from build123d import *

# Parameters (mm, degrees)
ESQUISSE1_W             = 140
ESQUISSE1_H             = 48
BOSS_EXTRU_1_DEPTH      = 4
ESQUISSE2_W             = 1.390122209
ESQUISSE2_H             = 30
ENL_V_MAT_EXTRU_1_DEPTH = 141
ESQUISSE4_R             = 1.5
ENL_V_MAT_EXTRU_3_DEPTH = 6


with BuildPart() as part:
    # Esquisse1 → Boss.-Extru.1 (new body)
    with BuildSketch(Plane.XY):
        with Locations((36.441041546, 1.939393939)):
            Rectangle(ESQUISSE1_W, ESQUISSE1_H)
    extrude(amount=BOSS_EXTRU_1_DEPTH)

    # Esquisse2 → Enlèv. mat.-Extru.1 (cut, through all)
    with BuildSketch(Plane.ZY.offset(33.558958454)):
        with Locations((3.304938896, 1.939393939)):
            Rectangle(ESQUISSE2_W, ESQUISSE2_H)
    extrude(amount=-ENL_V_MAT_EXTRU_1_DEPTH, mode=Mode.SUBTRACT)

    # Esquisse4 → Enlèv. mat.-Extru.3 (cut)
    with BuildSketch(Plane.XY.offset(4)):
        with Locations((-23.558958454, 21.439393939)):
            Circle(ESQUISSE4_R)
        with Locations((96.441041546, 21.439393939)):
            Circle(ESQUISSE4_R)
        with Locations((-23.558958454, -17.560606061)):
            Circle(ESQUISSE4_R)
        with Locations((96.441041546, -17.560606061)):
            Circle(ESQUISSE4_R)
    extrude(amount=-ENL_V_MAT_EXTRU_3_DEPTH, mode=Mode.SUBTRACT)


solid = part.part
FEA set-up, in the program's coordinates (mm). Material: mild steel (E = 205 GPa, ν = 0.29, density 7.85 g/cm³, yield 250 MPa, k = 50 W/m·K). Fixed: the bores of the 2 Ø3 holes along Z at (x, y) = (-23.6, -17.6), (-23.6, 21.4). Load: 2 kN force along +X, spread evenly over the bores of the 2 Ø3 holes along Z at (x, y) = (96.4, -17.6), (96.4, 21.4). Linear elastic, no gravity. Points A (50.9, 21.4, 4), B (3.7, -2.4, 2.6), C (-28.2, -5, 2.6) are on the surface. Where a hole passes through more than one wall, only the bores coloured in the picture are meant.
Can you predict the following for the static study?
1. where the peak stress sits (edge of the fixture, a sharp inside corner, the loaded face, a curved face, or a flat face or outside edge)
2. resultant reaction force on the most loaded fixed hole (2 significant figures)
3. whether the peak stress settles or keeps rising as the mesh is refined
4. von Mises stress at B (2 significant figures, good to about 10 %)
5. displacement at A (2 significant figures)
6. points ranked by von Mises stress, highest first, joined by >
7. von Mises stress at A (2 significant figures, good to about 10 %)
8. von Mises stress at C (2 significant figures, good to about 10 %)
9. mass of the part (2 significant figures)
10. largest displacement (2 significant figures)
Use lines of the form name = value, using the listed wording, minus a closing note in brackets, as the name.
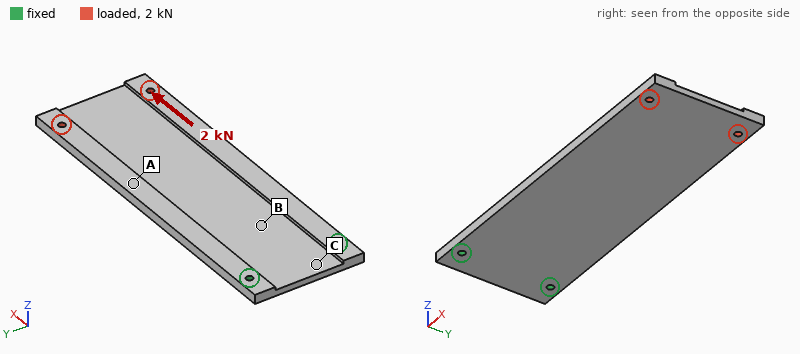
where the peak stress sits = edge of the fixture
resultant reaction force on the most loaded fixed hole = 1.0 kN
whether the peak stress settles or keeps rising as the mesh is refined = keeps rising
von Mises stress at B = 15 MPa
displacement at A = 0.050 mm
points ranked by von Mises stress, highest first, joined by > = A > B > C
von Mises stress at A = 24 MPa
von Mises stress at C = 5.4 MPa
mass of the part = 160 g
largest displacement = 0.16 mm
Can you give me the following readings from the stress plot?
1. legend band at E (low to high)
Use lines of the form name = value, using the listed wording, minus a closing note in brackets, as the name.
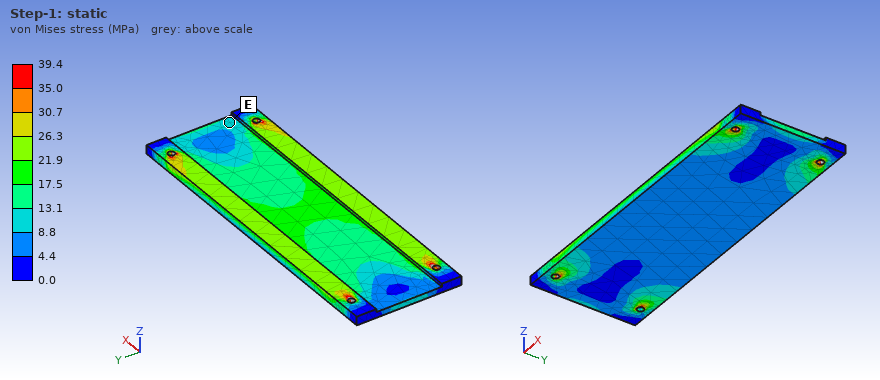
legend band at E = 8.8 to 13.1 MPa
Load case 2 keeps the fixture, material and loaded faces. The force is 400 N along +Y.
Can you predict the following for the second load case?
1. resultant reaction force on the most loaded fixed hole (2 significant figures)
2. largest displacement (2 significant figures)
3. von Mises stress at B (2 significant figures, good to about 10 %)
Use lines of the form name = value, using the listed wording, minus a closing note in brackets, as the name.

resultant reaction force on the most loaded fixed hole = 1.2 kN
largest displacement = 56 µm
von Mises stress at B = 12 MPa
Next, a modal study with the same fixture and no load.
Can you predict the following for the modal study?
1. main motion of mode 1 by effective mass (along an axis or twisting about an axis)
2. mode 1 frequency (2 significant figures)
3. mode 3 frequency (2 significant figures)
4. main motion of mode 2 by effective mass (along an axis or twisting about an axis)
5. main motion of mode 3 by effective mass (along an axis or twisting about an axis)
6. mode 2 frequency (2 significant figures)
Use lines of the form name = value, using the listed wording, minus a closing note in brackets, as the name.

main motion of mode 1 by effective mass = along Z
mode 1 frequency = 170 Hz
mode 3 frequency = 1100 Hz
main motion of mode 2 by effective mass = twisting about X
main motion of mode 3 by effective mass = along Z
mode 2 frequency = 840 Hz
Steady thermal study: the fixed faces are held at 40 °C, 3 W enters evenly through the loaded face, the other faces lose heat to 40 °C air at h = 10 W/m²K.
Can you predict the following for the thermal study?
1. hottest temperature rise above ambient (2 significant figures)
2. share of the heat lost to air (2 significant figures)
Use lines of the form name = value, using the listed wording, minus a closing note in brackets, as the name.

hottest temperature rise above ambient = 29 K
share of the heat lost to air = 61 %
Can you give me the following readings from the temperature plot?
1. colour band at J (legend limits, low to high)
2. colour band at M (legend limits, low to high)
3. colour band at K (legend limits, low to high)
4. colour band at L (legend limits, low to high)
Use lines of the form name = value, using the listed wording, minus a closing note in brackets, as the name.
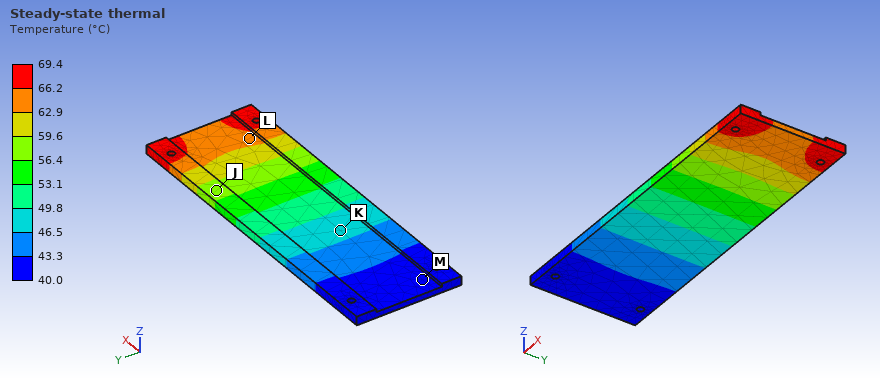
colour band at J = 56.4 to 59.6 °C
colour band at M = 40.0 to 43.3 °C
colour band at K = 46.5 to 49.8 °C
colour band at L = 62.9 to 66.2 °C
